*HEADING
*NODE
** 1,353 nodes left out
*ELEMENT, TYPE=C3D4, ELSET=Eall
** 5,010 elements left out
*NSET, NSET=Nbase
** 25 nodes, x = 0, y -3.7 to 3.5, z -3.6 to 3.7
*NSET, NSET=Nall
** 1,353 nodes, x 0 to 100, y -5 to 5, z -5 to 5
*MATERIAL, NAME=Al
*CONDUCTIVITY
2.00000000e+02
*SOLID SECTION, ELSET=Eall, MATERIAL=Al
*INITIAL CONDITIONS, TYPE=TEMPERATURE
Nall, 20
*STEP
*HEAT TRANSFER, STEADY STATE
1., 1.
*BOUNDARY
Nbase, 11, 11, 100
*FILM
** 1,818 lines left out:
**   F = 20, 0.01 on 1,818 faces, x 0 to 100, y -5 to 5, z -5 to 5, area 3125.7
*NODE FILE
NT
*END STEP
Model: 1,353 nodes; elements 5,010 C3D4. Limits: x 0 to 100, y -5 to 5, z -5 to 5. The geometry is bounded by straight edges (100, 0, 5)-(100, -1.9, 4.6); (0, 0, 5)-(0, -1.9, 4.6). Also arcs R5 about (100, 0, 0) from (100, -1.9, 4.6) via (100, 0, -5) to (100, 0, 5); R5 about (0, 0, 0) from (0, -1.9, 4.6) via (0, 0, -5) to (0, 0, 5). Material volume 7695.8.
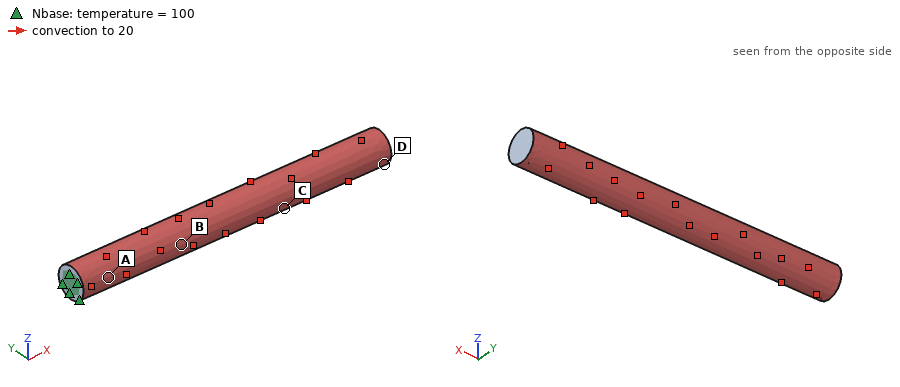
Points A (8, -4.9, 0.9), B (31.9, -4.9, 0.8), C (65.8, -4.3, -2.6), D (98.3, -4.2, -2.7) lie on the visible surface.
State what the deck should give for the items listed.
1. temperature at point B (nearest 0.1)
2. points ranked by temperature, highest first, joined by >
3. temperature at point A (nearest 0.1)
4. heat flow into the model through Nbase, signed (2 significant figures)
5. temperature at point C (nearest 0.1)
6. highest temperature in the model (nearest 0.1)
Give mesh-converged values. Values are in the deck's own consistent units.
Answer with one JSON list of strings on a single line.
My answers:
["95.9", "A > B > C > D", "98.8", "2300", "93.3", "100.0"]
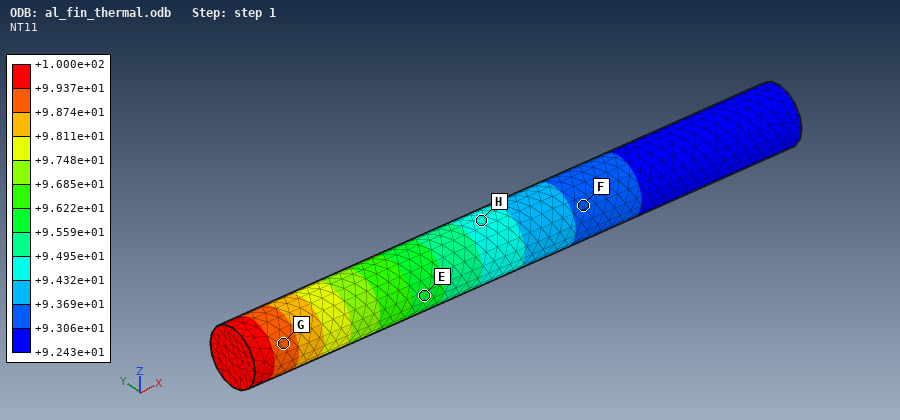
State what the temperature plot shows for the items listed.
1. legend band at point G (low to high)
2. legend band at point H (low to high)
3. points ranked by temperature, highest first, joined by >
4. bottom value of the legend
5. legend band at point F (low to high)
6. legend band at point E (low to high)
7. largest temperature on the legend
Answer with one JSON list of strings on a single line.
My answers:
["+9.874e+01 to +9.937e+01", "+9.432e+01 to +9.495e+01", "G > E > H > F", "+9.243e+01", "+9.306e+01 to +9.369e+01", "+9.559e+01 to +9.622e+01", "+1.000e+02"]
